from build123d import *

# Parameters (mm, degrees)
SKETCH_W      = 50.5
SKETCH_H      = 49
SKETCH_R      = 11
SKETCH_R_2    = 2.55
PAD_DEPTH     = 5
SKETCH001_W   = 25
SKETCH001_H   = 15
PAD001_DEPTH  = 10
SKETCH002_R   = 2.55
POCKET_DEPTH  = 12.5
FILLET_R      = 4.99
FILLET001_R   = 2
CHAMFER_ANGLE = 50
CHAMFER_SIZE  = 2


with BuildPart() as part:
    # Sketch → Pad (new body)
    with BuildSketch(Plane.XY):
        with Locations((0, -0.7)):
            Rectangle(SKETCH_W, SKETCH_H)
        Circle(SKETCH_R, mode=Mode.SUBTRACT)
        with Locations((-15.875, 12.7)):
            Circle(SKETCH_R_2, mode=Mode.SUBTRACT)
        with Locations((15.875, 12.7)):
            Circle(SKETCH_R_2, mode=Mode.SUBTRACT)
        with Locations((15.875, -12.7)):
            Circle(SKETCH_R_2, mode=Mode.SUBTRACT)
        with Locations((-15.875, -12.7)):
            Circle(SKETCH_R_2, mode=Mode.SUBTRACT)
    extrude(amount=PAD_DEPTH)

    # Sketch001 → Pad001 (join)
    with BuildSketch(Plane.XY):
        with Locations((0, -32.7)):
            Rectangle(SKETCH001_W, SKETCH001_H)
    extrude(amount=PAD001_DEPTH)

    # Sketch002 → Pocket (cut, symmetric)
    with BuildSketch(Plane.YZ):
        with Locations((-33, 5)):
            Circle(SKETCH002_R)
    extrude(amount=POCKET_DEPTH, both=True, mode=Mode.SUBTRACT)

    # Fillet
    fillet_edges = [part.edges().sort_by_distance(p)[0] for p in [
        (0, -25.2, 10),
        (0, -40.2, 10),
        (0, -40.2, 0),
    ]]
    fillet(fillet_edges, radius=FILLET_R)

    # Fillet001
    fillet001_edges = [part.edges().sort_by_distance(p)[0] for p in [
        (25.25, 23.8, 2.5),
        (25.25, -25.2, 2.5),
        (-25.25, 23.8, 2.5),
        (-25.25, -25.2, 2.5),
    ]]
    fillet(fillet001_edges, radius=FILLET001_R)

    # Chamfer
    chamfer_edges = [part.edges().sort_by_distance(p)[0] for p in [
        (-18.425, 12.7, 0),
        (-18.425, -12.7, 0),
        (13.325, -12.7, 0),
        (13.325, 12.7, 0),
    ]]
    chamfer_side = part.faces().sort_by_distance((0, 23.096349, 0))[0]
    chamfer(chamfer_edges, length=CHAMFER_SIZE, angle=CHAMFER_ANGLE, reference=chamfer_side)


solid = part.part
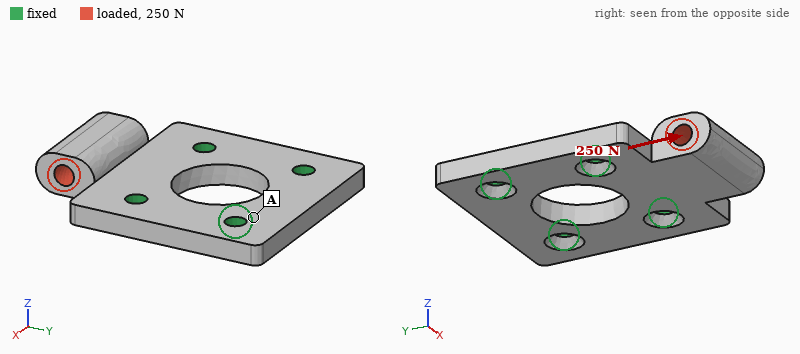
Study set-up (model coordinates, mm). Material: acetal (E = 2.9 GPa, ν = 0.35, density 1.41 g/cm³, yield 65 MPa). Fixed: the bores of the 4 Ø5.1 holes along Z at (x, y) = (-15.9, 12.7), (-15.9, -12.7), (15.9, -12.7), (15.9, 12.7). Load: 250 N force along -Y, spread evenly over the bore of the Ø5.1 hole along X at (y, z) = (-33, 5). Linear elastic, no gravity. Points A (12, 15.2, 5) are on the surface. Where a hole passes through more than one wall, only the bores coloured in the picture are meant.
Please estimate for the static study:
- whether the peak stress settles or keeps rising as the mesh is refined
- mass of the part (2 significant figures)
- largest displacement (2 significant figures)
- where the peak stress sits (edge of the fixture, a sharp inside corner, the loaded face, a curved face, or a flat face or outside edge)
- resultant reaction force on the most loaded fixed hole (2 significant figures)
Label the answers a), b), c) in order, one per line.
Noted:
a) keeps rising
b) 18 g
c) 0.22 mm
d) a sharp inside corner
e) 130 N
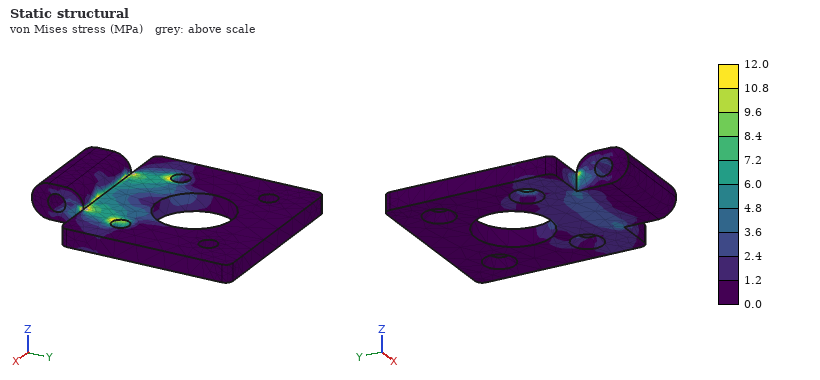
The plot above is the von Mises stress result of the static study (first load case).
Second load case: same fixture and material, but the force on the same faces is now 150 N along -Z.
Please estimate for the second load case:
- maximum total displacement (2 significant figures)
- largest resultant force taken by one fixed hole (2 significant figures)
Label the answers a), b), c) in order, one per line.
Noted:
a) 0.87 mm
b) 110 N
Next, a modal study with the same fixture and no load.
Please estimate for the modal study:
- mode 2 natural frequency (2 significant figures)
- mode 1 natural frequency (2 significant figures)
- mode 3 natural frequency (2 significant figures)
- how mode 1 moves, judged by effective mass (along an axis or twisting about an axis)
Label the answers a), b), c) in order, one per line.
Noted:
a) 4000 Hz
b) 1200 Hz
c) 4800 Hz
d) along Z
